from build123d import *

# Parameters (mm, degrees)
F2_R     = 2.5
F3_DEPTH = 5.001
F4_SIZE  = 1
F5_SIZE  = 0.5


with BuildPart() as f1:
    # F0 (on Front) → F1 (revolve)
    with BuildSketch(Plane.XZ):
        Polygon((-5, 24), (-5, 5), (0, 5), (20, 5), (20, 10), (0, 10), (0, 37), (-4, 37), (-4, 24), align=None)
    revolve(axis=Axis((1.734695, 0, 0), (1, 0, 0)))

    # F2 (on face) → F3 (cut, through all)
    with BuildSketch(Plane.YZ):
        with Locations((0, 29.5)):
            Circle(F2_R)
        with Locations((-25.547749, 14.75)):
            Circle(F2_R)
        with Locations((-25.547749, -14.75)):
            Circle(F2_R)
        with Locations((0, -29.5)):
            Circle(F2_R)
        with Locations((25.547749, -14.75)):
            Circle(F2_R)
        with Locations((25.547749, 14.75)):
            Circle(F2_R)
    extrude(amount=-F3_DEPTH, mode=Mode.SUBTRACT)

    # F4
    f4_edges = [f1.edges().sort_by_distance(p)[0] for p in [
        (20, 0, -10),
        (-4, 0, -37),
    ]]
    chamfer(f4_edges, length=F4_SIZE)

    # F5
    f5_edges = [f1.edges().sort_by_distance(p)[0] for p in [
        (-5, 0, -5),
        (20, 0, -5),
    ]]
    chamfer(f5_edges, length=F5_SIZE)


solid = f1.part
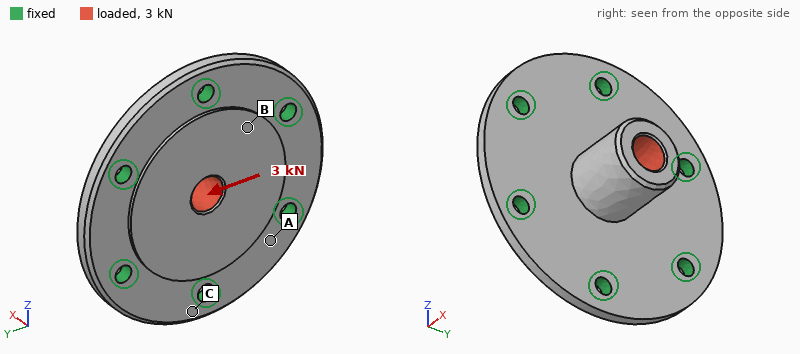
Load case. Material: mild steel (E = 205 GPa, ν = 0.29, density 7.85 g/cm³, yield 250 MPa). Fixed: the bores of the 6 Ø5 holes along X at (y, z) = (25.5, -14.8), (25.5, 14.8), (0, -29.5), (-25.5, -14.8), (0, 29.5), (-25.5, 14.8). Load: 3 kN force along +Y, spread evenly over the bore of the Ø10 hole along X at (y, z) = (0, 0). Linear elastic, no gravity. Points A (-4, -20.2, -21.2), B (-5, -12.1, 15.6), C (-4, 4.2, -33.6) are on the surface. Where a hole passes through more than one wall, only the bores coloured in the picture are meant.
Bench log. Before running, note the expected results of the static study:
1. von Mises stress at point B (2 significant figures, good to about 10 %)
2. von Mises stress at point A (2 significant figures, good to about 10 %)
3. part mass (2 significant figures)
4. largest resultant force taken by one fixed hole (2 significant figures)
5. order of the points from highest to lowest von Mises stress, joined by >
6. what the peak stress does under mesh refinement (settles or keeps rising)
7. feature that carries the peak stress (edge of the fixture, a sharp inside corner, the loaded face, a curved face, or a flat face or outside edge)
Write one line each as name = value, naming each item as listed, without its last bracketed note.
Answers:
von Mises stress at point B = 18 MPa
von Mises stress at point A = 10 MPa
part mass = 180 g
largest resultant force taken by one fixed hole = 730 N
order of the points from highest to lowest von Mises stress, joined by > = B > A > C
what the peak stress does under mesh refinement = keeps rising
feature that carries the peak stress = edge of the fixture
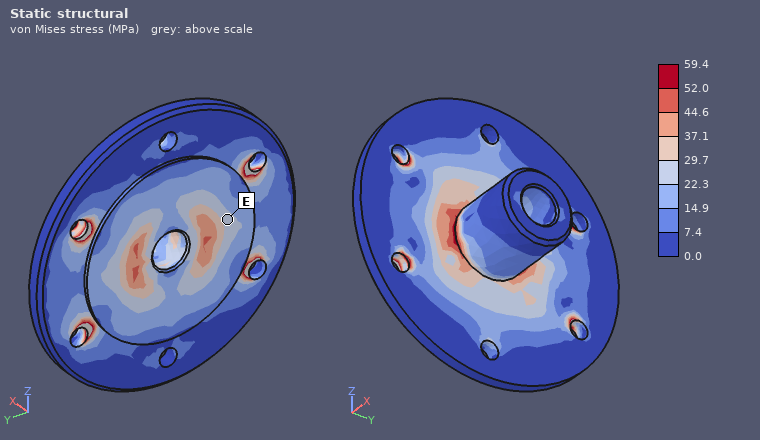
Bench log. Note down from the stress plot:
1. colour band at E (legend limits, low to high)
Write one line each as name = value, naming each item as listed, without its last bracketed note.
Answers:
colour band at E = 22.3 to 29.7 MPa
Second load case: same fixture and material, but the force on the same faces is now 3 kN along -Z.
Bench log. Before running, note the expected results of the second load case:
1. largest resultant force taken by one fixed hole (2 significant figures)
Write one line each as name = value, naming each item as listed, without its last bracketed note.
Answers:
largest resultant force taken by one fixed hole = 830 N
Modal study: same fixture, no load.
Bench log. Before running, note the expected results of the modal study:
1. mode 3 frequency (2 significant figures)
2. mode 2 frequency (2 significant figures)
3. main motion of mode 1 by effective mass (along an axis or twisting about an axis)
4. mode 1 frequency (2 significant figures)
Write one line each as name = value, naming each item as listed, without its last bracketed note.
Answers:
mode 3 frequency = 9900 Hz
mode 2 frequency = 9900 Hz
main motion of mode 1 by effective mass = along X
mode 1 frequency = 8400 Hz
